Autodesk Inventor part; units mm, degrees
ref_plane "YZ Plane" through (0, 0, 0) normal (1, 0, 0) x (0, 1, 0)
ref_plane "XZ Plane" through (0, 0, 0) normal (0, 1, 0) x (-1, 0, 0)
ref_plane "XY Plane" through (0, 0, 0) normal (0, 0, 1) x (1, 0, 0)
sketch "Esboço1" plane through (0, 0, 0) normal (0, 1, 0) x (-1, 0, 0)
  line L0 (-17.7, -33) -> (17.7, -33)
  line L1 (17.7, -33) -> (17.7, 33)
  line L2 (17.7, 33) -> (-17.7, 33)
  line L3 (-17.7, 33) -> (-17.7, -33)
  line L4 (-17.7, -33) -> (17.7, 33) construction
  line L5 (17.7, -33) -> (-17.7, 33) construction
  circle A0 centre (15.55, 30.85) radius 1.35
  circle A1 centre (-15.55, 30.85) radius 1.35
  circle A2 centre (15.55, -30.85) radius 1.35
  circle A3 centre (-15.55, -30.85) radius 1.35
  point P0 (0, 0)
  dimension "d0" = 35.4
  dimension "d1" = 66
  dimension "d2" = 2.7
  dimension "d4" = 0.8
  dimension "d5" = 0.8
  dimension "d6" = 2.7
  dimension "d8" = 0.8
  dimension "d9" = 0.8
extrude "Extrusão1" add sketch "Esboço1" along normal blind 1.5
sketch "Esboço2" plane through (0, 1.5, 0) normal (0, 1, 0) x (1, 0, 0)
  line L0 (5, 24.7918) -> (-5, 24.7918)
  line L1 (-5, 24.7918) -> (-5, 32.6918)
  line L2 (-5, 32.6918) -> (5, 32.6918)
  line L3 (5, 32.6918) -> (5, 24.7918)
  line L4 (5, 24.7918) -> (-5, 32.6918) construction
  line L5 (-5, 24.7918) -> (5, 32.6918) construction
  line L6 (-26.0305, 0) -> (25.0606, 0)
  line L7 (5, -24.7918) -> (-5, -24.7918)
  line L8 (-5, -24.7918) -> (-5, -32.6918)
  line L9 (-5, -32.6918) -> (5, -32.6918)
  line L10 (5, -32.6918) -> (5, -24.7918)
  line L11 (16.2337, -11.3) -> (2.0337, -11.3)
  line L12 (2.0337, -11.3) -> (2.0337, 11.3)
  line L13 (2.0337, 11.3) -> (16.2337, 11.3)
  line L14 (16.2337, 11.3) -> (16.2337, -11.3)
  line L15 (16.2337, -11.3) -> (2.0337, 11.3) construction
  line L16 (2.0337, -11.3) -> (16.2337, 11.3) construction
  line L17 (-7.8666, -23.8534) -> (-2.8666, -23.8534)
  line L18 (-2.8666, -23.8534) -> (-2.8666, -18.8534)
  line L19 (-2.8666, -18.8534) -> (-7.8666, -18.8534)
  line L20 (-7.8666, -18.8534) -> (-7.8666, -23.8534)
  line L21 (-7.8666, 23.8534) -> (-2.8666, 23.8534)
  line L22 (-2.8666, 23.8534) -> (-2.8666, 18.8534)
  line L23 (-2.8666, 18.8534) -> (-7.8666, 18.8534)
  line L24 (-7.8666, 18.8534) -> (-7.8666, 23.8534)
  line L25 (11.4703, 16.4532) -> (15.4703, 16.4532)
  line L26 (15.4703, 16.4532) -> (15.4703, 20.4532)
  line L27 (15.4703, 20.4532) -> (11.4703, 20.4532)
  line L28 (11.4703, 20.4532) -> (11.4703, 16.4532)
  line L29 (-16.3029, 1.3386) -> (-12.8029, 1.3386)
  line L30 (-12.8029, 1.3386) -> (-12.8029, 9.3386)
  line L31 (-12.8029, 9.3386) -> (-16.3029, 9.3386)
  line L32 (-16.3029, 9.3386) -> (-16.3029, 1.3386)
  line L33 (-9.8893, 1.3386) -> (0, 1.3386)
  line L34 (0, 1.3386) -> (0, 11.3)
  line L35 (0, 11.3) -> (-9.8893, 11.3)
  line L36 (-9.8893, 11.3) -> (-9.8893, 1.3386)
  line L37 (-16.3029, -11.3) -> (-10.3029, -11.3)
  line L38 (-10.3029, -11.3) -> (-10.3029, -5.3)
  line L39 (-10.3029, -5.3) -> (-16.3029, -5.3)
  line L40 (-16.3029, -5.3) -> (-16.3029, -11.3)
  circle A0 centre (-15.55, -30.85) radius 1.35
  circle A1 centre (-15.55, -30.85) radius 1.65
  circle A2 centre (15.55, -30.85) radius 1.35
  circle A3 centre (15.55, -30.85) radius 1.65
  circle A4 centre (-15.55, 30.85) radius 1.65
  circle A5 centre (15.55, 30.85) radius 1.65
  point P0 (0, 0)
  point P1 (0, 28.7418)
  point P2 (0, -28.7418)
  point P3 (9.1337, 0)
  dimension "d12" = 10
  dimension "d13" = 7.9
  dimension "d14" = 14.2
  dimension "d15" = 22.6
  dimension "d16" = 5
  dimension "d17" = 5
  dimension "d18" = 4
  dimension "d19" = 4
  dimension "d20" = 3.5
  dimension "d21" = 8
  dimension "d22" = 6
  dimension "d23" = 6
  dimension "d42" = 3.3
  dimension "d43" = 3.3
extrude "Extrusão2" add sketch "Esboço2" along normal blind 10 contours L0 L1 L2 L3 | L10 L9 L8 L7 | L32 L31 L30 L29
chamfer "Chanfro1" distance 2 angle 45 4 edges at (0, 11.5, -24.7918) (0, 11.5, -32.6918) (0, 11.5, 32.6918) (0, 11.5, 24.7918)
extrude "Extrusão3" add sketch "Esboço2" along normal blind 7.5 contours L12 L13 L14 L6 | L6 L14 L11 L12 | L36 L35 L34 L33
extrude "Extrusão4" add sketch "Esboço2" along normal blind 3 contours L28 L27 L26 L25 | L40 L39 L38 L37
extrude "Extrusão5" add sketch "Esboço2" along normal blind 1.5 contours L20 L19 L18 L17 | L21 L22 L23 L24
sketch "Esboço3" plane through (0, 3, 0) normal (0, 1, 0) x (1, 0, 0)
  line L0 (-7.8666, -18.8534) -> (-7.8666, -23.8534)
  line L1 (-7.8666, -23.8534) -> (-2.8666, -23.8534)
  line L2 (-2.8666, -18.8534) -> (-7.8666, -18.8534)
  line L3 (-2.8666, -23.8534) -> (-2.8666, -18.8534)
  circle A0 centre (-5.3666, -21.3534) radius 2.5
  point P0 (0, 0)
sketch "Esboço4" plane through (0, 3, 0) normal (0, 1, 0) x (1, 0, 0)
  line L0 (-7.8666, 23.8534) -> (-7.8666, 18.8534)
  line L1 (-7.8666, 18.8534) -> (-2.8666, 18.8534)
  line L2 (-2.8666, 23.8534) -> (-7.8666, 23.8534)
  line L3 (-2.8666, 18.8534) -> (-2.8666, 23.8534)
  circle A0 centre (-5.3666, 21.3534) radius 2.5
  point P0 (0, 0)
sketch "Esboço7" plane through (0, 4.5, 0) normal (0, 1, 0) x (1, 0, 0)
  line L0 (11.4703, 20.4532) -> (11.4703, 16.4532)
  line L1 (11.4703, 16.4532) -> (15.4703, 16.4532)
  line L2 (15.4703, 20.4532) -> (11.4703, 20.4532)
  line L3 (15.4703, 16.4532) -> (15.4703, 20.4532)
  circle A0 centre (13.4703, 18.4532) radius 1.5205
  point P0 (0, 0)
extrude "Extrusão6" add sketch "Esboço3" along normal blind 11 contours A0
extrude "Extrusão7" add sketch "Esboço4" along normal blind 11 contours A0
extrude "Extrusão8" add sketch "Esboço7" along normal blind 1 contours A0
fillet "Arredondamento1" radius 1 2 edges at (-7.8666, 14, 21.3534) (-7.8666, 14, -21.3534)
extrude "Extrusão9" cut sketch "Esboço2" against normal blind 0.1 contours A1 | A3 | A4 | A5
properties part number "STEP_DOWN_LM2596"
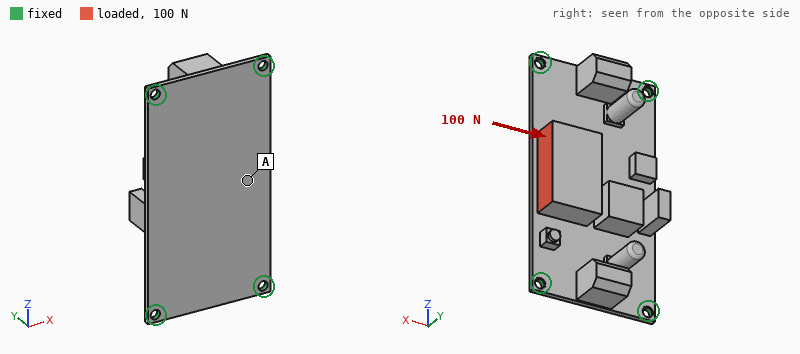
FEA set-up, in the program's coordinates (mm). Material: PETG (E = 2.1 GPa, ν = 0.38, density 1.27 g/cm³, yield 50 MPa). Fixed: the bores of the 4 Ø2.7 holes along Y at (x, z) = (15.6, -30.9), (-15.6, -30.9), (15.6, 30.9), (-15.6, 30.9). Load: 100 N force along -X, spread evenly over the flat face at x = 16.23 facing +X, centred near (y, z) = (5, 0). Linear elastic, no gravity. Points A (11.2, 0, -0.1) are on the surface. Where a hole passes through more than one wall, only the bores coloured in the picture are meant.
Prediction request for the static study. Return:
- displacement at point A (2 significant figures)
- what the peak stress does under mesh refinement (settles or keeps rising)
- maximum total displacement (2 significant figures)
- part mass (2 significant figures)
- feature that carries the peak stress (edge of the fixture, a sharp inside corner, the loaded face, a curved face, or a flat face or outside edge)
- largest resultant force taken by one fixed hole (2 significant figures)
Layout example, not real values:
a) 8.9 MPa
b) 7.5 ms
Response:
a) 0.40 mm
b) keeps rising
c) 0.89 mm
d) 12 g
e) edge of the fixture
f) 39 N
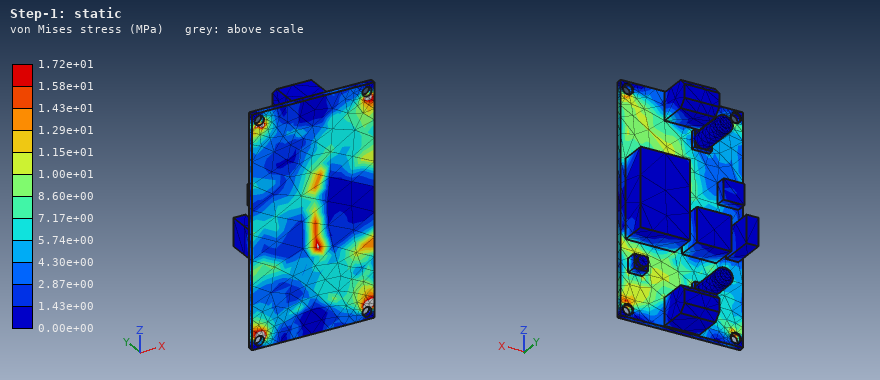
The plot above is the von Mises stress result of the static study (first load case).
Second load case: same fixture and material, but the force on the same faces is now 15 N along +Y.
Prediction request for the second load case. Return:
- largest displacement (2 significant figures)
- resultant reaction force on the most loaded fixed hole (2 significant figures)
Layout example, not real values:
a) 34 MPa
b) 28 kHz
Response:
a) 0.69 mm
b) 9.9 N
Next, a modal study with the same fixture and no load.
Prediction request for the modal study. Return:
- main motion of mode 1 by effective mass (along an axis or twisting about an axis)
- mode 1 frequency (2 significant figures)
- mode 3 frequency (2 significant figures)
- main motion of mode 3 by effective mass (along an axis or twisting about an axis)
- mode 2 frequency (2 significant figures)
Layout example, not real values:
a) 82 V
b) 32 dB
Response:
a) along Y
b) 370 Hz
c) 900 Hz
d) twisting about X
e) 580 Hz
